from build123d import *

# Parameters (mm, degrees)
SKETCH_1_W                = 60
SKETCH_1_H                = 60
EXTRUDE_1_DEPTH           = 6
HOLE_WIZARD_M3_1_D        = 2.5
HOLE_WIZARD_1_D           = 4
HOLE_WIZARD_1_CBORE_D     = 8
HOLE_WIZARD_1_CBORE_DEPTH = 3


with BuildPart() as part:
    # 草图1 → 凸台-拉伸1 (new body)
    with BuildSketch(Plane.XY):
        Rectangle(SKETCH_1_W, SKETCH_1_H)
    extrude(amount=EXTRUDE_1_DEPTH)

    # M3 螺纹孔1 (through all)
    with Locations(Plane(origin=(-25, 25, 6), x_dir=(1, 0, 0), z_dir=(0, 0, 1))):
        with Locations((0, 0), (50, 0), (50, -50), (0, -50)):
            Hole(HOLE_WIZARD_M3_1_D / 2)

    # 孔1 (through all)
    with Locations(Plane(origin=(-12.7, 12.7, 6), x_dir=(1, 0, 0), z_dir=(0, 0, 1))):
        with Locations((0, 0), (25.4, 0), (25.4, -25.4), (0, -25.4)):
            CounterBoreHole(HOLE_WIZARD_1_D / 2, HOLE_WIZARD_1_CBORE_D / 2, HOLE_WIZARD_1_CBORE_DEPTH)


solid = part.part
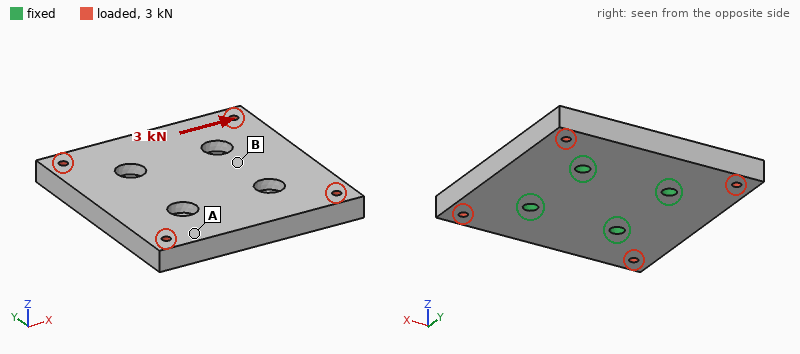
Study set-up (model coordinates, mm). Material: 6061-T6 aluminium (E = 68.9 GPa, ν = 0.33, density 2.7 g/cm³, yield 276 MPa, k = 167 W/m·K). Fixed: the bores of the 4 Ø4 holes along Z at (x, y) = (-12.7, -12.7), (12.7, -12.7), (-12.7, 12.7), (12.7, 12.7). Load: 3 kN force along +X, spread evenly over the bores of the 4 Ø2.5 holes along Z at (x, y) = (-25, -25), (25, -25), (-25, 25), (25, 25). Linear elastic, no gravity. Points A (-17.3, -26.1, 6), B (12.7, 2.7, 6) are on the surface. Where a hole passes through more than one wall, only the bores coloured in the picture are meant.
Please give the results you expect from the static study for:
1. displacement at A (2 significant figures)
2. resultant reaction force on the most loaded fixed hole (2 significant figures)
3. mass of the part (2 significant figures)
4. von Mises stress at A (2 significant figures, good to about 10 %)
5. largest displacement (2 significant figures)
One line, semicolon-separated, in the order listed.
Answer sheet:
4.7 µm; 760 N; 56 g; 10 MPa; 7.4 µm
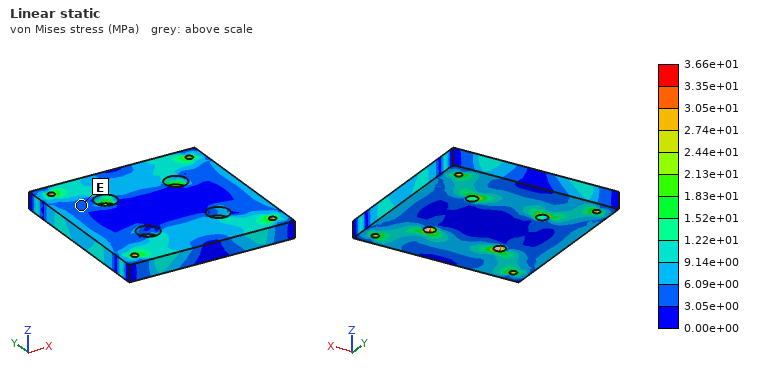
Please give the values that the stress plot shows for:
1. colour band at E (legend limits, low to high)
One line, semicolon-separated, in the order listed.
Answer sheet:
3.05e+00 to 6.09e+00 MPa
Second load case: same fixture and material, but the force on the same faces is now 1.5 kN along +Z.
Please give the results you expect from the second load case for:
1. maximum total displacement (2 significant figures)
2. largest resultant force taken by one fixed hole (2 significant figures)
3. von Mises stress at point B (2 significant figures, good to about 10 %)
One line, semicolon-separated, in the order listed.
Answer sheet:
51 µm; 690 N; 14 MPa
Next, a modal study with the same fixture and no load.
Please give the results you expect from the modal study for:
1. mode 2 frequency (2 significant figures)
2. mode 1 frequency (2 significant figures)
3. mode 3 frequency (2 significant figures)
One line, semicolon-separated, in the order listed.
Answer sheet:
9400 Hz; 9400 Hz; 9500 Hz
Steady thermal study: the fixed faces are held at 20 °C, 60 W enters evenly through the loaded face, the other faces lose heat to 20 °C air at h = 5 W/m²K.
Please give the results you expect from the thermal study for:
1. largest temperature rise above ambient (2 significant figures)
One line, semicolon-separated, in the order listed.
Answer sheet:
19 K
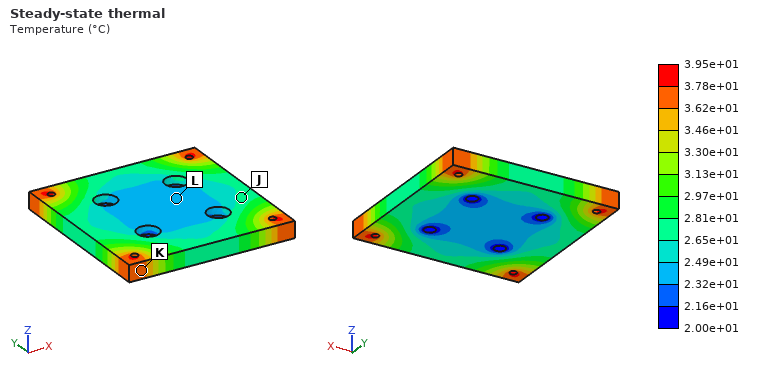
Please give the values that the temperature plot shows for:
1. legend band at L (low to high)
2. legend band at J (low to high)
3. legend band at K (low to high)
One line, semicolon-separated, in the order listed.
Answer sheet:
2.32e+01 to 2.49e+01 °C; 2.65e+01 to 2.81e+01 °C; 3.62e+01 to 3.78e+01 °C
